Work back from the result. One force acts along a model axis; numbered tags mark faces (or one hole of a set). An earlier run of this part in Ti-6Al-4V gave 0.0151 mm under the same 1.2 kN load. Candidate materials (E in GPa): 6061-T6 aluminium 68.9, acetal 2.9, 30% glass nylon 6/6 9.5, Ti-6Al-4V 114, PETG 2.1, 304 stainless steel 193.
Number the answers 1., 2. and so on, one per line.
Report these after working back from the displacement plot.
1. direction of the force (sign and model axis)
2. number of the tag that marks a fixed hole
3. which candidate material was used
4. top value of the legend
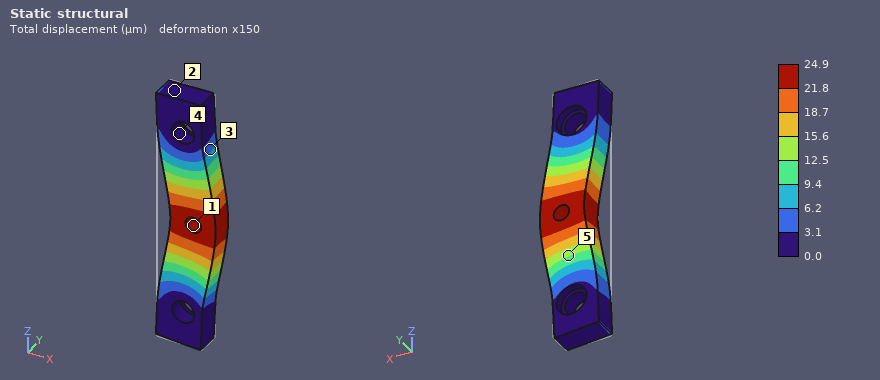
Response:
1. +X
2. 4
3. 6061-T6 aluminium
4. 24.9 µm
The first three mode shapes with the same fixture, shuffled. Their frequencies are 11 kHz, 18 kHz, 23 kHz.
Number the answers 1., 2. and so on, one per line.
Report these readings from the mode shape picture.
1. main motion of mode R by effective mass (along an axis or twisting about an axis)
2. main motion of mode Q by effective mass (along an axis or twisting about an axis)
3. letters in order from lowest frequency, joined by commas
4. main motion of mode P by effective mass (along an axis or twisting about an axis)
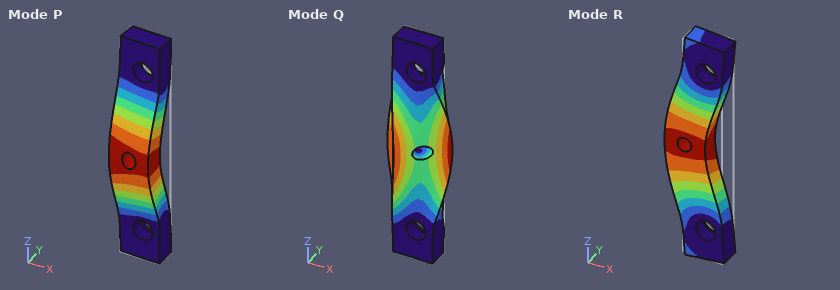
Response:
1. along X
2. twisting about Z
3. P, R, Q
4. along Y
